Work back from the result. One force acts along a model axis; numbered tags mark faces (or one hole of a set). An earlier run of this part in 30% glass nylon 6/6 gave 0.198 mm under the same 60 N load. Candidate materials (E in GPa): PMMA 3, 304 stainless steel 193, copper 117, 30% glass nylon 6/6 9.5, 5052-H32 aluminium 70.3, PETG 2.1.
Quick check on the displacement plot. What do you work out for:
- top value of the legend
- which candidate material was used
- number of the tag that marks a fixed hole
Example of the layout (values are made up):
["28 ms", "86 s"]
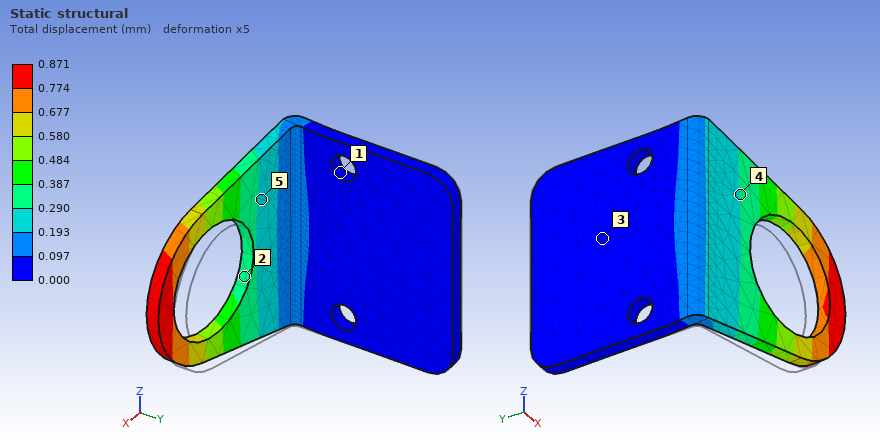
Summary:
["0.871 mm", "PETG", "1"]
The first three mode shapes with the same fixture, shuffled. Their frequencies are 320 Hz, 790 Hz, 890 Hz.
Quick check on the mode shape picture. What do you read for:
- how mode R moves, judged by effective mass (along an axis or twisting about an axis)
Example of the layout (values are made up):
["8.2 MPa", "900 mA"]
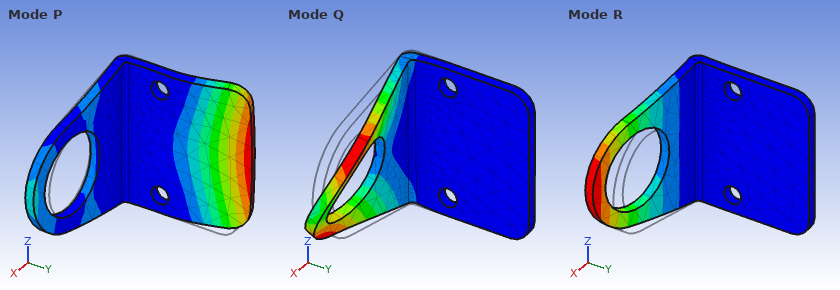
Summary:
["along Y"]
